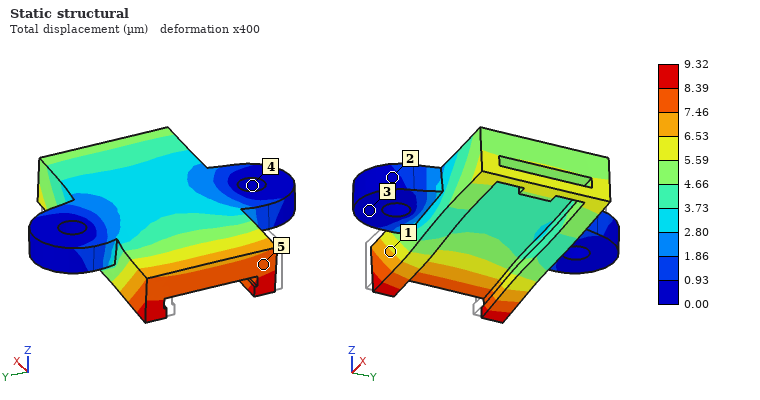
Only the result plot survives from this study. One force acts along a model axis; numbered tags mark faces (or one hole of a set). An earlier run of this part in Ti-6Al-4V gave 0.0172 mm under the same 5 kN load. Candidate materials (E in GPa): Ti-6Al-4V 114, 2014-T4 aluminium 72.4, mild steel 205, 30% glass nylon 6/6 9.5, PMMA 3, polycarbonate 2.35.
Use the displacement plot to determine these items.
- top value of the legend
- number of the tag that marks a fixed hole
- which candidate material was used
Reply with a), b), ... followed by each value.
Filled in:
a) 9.32 µm
b) 4
c) mild steel
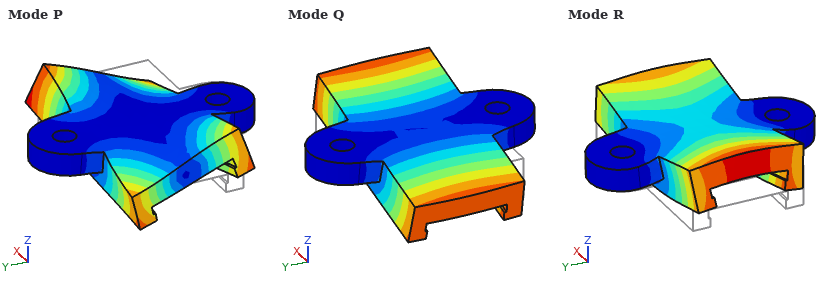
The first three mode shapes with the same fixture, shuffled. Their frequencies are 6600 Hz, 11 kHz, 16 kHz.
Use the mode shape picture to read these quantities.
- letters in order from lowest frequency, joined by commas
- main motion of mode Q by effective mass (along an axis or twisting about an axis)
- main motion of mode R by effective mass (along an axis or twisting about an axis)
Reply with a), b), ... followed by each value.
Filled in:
a) Q, R, P
b) twisting about Y
c) along Z
